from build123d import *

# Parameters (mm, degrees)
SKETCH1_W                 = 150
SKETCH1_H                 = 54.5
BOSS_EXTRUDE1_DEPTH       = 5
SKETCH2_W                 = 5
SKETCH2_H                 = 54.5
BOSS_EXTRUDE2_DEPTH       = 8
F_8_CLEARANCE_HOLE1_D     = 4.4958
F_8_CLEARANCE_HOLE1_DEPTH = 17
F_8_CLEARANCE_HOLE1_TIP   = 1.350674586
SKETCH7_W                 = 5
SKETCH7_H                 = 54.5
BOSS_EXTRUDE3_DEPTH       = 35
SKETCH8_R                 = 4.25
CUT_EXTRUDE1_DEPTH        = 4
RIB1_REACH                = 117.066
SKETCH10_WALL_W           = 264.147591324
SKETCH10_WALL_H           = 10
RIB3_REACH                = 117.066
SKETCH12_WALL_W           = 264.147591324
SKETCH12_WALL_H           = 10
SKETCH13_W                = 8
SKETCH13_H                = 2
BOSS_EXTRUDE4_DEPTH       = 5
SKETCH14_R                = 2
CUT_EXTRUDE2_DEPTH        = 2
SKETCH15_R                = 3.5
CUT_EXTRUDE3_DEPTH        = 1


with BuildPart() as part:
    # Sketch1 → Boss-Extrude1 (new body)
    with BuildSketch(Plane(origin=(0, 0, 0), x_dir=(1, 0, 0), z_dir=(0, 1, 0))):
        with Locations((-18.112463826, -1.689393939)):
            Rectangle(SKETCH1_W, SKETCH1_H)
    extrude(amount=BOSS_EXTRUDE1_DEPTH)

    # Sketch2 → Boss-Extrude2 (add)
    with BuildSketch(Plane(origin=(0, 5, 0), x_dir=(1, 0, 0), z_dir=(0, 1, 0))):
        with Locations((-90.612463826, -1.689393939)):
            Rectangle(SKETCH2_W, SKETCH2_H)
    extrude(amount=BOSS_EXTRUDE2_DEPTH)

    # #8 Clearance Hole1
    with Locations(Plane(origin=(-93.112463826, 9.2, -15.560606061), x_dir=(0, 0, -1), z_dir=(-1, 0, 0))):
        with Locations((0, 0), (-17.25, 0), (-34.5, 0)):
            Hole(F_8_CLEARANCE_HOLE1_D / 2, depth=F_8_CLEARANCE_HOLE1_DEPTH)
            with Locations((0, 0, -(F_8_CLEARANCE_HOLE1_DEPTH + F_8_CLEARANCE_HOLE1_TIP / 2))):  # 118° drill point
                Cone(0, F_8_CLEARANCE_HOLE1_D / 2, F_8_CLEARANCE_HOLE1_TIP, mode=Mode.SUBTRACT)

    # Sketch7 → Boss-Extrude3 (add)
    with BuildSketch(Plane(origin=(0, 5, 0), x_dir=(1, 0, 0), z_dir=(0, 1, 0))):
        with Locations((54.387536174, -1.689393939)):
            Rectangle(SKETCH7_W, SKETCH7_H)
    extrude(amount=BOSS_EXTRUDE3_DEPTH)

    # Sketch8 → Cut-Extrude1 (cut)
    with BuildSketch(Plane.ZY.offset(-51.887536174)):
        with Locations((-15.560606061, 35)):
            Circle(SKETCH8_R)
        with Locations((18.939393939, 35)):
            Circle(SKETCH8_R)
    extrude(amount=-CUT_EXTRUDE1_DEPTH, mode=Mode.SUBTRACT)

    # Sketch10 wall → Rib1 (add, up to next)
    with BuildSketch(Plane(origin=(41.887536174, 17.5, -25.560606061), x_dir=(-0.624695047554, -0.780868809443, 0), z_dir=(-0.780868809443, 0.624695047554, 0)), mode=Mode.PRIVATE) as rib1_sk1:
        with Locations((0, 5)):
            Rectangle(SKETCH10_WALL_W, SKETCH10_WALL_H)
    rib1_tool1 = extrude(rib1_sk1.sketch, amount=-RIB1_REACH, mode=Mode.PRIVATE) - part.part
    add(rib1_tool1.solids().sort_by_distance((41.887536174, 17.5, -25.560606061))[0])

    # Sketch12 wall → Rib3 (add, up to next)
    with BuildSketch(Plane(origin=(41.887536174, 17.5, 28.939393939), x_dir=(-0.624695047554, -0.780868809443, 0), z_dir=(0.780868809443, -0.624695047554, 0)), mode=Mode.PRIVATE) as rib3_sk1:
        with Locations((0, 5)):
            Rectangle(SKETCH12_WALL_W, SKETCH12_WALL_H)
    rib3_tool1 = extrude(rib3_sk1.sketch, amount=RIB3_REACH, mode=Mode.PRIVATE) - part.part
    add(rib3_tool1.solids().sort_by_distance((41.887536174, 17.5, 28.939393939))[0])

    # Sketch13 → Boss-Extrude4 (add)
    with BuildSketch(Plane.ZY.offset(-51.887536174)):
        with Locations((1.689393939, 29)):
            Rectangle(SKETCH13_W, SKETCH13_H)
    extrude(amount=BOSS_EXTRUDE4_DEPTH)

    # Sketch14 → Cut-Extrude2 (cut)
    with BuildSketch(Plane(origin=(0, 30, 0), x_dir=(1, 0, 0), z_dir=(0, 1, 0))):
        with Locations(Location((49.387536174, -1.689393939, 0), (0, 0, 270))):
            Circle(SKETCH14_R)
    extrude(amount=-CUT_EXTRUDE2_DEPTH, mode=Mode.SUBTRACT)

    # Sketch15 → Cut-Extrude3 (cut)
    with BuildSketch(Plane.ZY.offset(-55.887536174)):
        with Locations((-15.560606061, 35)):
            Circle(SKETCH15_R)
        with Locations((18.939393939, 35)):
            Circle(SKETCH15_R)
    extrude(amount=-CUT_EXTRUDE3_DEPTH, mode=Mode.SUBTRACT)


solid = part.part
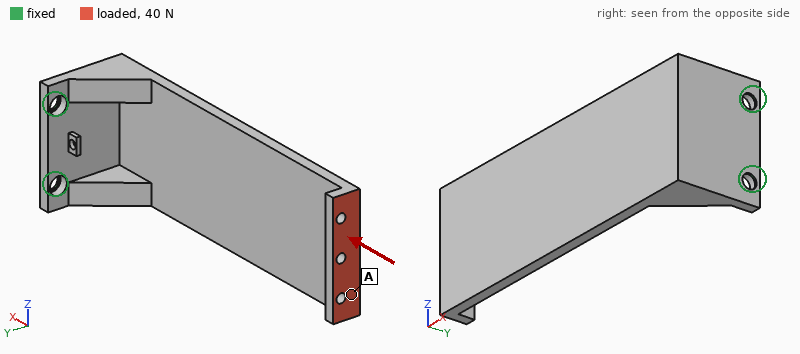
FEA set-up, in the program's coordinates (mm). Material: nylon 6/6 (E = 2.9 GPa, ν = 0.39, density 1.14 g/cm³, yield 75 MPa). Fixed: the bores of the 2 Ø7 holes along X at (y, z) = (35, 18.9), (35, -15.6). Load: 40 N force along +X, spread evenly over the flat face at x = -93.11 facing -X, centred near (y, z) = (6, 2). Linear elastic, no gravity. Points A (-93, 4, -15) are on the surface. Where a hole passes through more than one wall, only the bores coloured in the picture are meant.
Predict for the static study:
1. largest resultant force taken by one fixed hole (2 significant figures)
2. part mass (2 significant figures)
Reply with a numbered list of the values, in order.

1. 21 N
2. 65 g
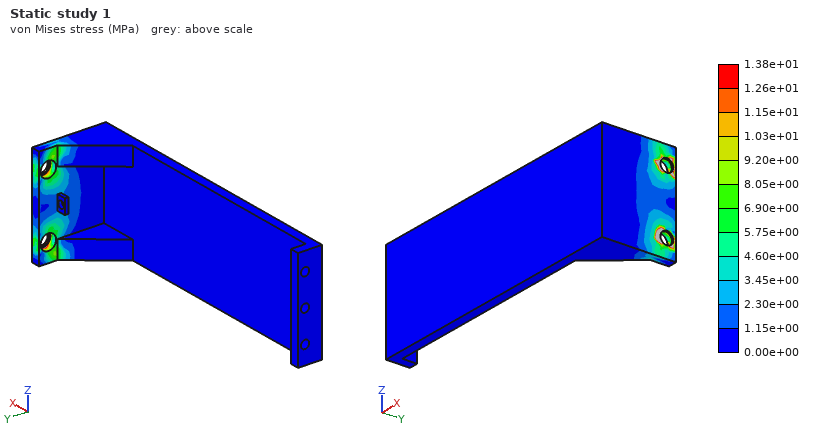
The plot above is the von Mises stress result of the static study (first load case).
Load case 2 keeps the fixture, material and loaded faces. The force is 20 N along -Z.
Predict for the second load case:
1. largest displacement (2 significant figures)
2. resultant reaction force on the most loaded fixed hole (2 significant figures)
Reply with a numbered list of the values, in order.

1. 1.8 mm
2. 78 N
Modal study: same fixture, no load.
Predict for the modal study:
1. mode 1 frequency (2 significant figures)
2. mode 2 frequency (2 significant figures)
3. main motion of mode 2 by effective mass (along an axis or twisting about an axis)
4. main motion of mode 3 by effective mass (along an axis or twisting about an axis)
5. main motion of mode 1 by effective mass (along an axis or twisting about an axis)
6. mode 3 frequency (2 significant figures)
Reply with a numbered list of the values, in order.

1. 46 Hz
2. 130 Hz
3. along Z
4. along X
5. along Y
6. 210 Hz
